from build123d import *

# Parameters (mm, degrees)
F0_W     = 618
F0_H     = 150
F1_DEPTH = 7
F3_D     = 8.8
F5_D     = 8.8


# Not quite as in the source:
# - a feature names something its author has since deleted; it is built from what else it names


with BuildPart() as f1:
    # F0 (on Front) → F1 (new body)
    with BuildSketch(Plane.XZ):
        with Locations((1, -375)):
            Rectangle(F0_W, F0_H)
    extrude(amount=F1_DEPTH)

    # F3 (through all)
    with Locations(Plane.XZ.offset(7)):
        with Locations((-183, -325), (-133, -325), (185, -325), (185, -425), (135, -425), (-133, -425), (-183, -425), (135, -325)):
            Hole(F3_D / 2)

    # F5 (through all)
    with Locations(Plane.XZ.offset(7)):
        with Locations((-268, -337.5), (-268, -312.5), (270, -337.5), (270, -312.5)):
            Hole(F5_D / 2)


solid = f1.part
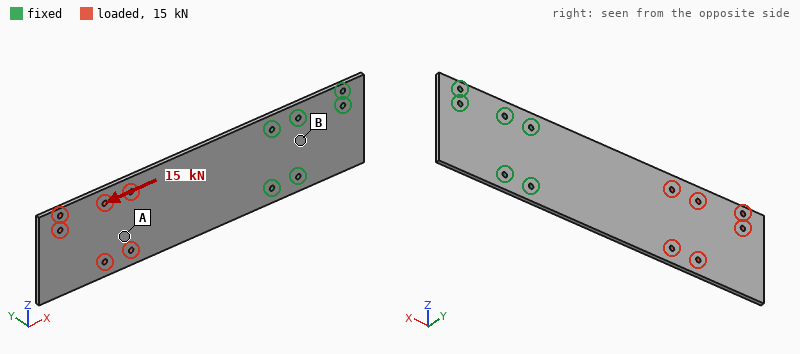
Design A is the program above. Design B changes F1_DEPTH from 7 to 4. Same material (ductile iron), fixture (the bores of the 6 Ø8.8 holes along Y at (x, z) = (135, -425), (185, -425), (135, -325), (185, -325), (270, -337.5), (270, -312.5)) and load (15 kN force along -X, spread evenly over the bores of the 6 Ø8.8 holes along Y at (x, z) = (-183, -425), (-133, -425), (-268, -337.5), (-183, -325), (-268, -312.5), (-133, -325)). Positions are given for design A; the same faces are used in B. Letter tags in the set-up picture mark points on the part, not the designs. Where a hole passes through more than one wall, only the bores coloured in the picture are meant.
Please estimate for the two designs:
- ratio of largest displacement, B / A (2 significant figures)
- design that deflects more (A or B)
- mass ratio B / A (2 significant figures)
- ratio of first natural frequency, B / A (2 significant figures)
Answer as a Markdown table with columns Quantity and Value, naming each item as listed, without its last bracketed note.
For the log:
| Quantity | Value |
|---|---|
| ratio of largest displacement, B / A | 1.8 |
| design that deflects more | B |
| mass ratio B / A | 0.57 |
| ratio of first natural frequency, B / A | 0.57 |
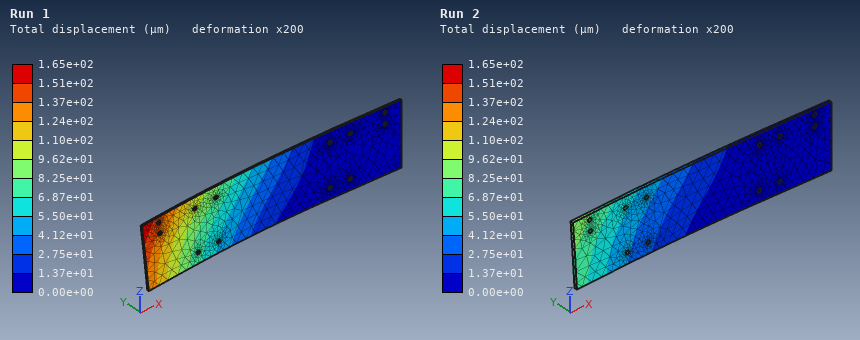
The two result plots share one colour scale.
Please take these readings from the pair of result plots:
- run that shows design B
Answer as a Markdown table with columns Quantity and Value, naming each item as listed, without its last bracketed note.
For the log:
| Quantity | Value |
|---|---|
| run that shows design B | Run 1 |
